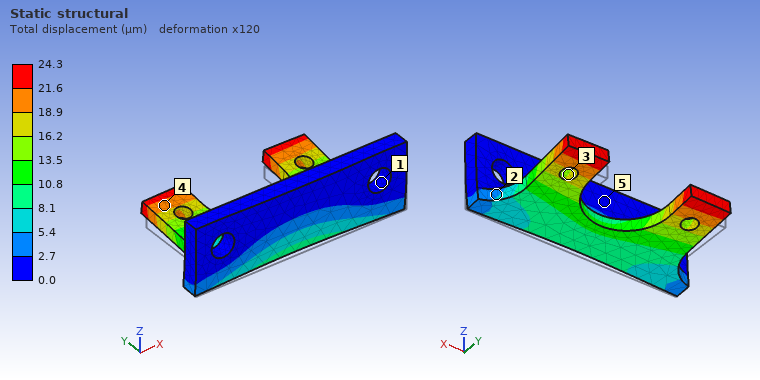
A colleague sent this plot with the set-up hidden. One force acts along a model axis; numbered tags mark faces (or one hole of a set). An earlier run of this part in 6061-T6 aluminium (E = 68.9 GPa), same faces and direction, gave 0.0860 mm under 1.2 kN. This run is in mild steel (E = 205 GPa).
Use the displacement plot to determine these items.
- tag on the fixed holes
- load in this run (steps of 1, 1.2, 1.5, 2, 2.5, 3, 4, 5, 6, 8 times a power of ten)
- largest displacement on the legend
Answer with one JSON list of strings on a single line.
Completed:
["1", "1 kN", "24.3 µm"]
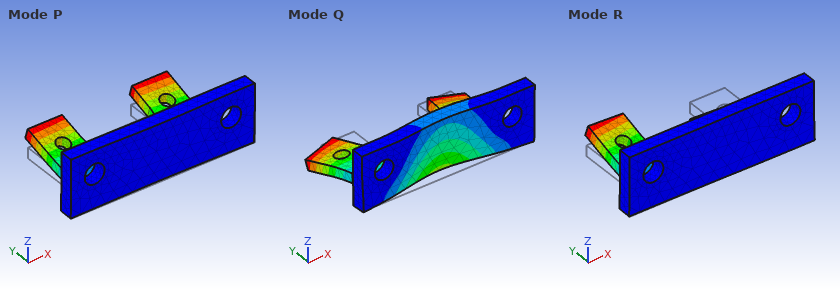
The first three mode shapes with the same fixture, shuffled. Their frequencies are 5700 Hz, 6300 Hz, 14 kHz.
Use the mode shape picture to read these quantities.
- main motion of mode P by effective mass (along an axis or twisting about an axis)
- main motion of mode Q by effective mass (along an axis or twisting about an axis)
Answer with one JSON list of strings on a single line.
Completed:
["along Z", "along Y"]
